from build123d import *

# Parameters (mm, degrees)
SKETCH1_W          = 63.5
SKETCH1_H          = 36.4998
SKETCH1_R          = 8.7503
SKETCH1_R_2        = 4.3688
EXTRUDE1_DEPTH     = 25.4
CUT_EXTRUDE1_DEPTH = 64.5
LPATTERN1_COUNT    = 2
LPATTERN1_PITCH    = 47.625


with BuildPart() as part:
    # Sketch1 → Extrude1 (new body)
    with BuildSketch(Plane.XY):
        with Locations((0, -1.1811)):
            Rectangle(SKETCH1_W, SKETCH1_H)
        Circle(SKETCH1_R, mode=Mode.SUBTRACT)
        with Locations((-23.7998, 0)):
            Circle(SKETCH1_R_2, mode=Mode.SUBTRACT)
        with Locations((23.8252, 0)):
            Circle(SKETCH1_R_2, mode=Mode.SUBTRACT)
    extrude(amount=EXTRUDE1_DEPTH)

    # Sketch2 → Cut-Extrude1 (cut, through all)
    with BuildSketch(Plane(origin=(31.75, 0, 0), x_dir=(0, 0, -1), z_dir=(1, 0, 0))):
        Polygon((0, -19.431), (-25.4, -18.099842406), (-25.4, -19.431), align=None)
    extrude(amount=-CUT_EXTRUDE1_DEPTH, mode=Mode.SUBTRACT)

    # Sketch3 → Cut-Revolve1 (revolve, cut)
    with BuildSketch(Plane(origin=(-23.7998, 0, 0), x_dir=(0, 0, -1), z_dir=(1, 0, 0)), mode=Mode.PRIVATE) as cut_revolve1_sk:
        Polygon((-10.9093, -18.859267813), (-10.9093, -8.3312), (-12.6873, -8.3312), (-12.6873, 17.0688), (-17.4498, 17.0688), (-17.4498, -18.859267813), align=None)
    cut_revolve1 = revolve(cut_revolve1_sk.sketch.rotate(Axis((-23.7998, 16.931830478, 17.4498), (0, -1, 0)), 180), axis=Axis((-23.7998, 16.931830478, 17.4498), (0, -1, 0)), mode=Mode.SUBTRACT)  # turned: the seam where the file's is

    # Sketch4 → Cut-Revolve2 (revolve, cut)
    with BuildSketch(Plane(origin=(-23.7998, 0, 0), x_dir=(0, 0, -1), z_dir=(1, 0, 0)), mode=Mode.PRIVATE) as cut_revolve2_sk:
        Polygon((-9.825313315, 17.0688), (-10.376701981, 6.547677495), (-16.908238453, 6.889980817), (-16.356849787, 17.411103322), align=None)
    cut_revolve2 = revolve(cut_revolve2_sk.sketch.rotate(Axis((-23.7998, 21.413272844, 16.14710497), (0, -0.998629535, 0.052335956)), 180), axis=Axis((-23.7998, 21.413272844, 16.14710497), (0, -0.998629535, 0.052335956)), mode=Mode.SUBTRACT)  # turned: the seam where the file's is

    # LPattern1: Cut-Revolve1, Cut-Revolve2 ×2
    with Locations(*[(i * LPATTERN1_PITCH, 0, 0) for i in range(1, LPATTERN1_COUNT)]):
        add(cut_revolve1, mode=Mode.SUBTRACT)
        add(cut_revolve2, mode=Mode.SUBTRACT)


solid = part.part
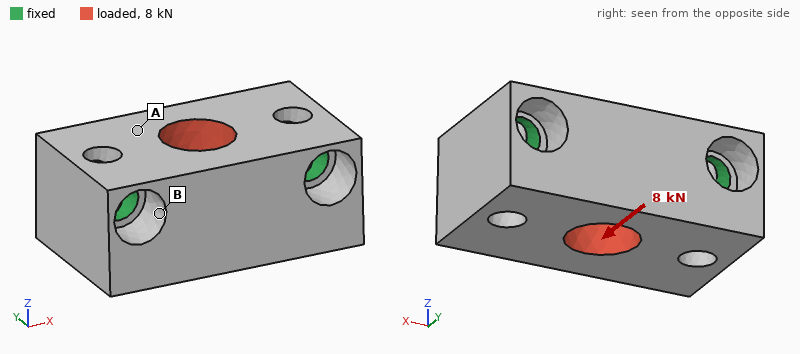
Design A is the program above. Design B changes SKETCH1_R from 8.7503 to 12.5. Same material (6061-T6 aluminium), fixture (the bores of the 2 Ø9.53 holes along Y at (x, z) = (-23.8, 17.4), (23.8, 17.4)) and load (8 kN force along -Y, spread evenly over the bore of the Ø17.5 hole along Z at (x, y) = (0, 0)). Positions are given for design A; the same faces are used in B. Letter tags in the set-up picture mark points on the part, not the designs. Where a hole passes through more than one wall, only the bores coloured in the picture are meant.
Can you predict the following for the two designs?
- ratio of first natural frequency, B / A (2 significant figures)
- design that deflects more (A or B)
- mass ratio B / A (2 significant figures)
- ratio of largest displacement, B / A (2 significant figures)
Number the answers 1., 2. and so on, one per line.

1. 1.0
2. B
3. 0.85
4. 1.2
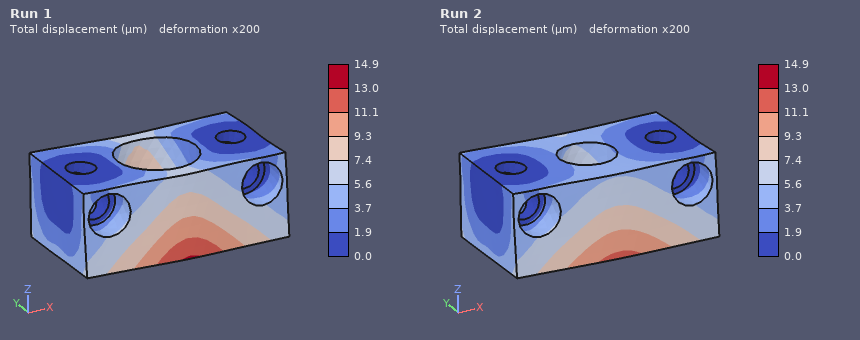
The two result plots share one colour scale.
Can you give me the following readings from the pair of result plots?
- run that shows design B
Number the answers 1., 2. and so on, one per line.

1. Run 1
